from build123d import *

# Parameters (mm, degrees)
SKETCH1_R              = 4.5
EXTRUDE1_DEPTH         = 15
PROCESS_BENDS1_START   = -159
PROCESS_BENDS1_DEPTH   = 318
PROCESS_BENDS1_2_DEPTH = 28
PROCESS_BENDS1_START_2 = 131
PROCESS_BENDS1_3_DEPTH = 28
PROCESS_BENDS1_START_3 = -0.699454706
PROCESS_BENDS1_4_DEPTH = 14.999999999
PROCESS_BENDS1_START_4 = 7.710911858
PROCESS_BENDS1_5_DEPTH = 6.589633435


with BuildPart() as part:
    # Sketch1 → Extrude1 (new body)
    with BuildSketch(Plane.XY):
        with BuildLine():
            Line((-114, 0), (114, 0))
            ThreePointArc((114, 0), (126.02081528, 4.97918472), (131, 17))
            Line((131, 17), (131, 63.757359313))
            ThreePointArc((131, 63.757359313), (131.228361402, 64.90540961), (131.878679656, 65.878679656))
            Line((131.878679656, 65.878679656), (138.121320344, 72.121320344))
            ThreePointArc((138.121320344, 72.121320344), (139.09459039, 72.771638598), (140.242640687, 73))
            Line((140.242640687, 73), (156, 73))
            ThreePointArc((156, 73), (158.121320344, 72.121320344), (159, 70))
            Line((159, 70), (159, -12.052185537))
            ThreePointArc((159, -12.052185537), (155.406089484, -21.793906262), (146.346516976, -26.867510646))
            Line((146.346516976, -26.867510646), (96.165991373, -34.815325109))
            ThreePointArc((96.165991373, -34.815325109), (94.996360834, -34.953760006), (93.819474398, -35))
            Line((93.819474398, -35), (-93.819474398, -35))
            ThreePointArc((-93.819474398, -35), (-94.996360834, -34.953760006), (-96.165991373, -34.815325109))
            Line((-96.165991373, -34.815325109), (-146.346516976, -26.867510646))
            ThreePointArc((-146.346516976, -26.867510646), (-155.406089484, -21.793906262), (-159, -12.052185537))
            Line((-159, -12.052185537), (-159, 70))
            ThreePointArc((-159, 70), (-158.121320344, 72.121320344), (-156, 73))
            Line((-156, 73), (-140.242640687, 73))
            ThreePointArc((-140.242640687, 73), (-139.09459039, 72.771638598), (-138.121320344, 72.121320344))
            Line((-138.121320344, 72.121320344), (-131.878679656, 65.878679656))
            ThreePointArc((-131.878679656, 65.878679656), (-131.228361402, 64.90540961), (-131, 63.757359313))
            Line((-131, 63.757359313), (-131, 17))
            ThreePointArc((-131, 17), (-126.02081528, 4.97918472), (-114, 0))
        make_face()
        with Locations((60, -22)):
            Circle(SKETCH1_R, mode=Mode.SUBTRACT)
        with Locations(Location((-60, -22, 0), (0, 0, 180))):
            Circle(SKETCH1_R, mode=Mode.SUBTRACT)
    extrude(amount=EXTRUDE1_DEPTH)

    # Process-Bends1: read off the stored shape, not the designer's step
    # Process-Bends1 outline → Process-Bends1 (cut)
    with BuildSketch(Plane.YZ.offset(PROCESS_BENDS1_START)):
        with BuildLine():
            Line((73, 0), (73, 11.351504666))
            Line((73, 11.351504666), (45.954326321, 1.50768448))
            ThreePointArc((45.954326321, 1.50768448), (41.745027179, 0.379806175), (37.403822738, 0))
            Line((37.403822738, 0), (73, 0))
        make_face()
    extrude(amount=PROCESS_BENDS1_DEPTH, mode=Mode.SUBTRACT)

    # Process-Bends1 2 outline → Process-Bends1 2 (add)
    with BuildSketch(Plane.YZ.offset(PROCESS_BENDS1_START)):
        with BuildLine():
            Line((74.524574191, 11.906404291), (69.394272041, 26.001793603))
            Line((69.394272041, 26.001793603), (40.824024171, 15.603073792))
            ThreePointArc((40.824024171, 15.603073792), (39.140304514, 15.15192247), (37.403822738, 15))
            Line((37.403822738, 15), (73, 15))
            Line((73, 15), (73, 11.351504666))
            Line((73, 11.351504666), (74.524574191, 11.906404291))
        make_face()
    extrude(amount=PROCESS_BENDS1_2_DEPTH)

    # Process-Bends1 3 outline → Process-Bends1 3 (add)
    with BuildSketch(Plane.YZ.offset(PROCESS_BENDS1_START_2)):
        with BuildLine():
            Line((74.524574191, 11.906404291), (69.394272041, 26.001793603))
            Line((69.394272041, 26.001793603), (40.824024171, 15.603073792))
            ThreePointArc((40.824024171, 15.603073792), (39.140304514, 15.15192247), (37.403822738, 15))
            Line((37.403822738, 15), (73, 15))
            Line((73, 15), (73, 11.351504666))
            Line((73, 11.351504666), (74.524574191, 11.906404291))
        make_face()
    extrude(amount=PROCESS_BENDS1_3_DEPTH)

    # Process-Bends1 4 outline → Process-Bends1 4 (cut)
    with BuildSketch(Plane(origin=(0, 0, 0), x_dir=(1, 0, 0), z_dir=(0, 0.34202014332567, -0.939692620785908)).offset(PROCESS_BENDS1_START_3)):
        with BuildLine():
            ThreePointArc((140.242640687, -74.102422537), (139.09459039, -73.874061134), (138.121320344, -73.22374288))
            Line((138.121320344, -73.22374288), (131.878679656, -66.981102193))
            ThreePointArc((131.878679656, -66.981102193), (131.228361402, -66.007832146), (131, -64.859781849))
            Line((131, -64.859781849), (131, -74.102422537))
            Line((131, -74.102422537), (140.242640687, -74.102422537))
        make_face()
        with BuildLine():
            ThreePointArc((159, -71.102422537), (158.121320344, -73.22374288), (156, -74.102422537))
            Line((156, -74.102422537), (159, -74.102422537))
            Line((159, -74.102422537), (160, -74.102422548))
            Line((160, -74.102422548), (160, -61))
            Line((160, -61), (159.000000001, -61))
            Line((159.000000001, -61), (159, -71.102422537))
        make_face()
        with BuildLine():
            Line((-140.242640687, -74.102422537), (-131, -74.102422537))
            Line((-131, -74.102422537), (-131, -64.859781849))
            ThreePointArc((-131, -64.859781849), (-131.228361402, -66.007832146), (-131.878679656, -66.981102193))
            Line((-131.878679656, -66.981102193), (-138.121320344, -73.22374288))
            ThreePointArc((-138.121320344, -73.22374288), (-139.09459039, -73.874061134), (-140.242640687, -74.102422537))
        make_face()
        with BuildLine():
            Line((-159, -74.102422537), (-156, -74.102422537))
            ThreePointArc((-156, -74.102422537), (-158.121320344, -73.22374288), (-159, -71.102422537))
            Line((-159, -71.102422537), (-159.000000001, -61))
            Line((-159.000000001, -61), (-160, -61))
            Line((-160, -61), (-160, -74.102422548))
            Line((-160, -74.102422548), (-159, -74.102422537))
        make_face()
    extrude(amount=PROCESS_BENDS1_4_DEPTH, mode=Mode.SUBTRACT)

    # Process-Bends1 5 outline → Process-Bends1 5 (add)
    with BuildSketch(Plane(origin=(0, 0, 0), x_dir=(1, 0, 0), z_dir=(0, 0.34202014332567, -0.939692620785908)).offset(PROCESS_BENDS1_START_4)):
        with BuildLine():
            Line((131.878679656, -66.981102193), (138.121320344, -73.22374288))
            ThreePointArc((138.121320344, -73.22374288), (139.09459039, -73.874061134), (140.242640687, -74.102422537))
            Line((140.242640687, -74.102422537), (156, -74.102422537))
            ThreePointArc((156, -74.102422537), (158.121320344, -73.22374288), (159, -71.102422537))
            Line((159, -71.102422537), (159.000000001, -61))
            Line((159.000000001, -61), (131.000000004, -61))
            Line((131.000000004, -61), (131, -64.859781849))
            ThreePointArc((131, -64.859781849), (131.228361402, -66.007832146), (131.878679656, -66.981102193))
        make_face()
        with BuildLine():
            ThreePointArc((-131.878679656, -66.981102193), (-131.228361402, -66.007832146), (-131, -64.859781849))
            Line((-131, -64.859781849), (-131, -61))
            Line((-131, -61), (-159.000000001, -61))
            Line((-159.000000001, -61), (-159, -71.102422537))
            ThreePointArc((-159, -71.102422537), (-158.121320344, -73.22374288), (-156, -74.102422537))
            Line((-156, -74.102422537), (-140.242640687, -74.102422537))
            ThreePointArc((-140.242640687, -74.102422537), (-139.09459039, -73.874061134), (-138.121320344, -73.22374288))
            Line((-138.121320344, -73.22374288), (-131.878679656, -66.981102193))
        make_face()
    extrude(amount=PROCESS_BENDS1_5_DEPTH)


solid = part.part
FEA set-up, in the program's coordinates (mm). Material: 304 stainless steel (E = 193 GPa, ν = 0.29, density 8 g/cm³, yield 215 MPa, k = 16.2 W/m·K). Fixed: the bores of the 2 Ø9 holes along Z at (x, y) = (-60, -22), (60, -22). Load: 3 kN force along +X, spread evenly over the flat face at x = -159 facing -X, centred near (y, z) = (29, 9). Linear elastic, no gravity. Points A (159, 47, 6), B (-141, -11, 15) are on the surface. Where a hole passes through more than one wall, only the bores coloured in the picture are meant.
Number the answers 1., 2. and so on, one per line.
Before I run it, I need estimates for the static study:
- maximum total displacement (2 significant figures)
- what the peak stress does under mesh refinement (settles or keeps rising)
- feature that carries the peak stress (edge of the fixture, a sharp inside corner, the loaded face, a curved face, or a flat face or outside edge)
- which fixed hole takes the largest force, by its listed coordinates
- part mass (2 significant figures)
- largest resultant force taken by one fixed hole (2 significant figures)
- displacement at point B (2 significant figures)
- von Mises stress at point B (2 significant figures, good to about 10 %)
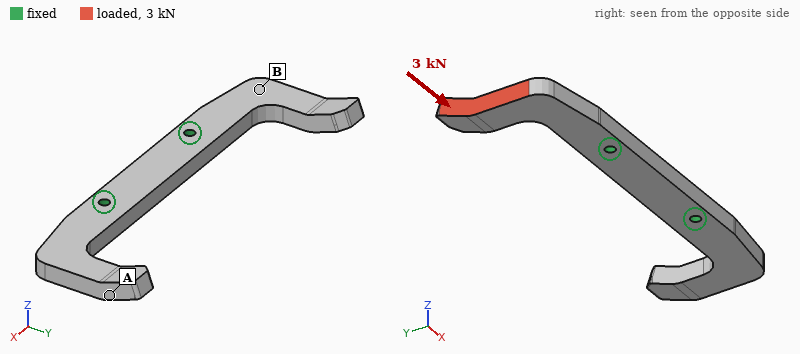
1. 0.19 mm
2. keeps rising
3. edge of the fixture
4. (-60, -22)
5. 1.7 kg
6. 1.8 kN
7. 0.069 mm
8. 18 MPa
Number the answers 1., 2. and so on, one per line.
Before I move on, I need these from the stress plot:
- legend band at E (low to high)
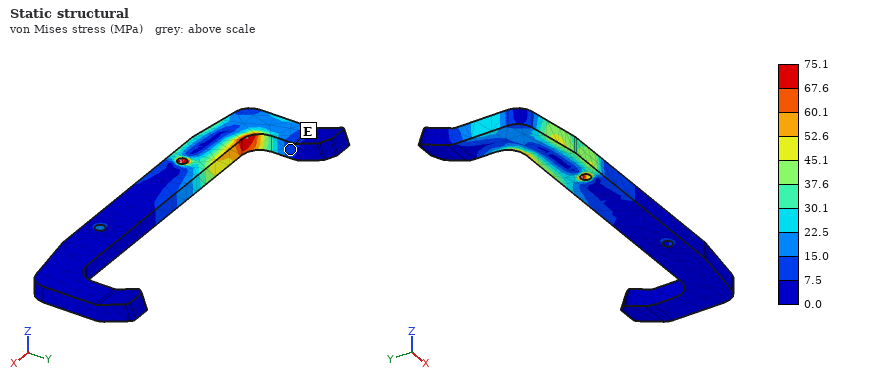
1. 7.5 to 15.0 MPa
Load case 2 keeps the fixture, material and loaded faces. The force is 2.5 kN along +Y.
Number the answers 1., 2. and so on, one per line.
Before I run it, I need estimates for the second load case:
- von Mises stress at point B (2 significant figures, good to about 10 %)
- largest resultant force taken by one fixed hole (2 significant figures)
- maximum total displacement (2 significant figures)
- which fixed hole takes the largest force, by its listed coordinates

1. 18 MPa
2. 4.1 kN
3. 0.21 mm
4. (-60, -22)
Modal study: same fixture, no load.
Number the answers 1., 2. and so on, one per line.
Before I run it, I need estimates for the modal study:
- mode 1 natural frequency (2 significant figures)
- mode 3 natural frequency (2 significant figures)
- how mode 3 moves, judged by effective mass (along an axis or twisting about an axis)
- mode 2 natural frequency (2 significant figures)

1. 600 Hz
2. 1100 Hz
3. along Y
4. 600 Hz
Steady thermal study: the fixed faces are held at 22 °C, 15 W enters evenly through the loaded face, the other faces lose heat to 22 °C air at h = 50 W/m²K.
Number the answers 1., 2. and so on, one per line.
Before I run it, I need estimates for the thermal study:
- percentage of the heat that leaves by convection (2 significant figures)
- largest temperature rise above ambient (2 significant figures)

1. 92 %
2. 45 K
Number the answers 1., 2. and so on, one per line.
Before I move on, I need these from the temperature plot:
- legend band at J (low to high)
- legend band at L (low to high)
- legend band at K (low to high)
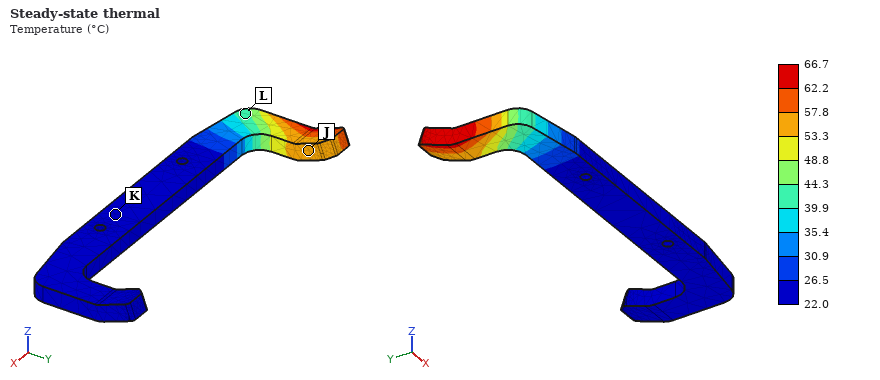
1. 53.3 to 57.8 °C
2. 39.9 to 44.3 °C
3. 22.0 to 26.5 °C
